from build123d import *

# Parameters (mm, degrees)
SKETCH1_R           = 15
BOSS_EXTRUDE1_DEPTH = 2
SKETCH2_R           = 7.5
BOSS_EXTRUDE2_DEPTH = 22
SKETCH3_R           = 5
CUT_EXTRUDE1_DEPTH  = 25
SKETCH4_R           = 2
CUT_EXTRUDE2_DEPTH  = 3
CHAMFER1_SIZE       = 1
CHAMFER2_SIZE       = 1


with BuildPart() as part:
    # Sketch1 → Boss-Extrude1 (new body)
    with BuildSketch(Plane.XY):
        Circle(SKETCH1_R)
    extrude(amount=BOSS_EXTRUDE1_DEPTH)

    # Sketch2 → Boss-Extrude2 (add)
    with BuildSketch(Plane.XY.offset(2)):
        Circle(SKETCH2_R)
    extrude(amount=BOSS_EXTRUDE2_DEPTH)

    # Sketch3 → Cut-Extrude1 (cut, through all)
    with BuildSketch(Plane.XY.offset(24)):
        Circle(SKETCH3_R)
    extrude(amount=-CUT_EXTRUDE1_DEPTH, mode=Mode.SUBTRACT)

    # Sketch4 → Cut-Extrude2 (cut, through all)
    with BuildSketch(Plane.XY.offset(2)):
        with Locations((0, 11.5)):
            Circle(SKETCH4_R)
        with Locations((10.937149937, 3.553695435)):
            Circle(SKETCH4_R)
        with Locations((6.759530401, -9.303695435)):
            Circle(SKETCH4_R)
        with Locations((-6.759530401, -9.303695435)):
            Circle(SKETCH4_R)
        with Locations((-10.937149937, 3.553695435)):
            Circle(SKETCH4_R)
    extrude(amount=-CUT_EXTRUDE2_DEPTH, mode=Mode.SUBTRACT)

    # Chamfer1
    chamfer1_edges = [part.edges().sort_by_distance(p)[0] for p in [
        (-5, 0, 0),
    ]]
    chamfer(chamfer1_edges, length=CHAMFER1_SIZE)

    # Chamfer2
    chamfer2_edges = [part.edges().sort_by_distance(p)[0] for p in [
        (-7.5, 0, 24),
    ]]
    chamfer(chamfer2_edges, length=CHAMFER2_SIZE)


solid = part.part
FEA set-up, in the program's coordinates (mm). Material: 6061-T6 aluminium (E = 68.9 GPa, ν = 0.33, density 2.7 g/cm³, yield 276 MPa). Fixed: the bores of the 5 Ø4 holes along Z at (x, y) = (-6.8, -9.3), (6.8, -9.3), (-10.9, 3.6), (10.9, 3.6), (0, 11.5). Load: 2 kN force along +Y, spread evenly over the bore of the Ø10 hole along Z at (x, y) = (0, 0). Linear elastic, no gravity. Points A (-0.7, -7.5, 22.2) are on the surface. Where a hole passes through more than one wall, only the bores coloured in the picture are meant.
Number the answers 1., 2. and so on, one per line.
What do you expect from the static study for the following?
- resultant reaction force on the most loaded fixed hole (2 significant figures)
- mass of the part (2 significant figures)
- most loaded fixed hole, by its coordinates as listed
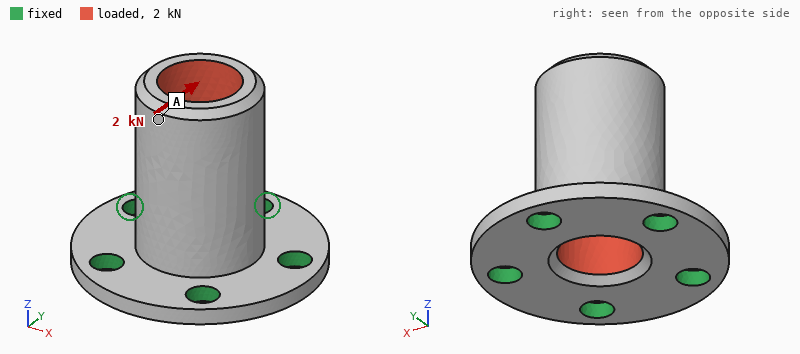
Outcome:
1. 1.2 kN
2. 8.8 g
3. (0, 11.5)
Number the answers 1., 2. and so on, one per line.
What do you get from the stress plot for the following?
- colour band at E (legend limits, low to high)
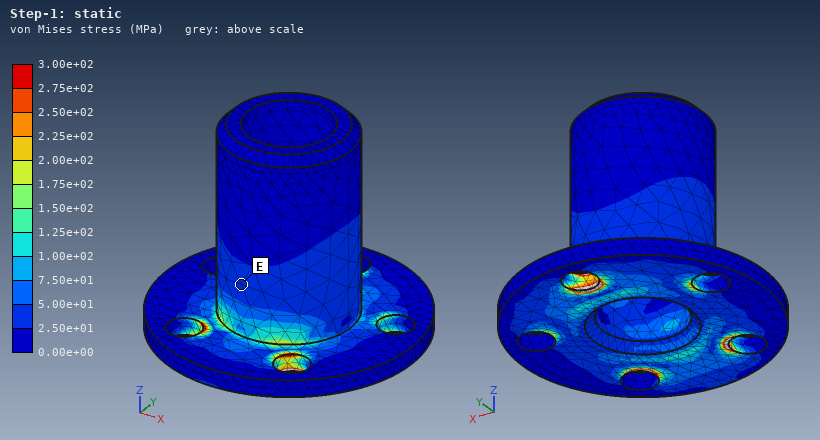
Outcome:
1. 2.50e+01 to 5.00e+01 MPa
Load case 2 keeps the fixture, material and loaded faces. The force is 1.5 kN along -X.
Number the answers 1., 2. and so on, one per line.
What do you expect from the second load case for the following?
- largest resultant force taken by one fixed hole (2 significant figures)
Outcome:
1. 850 N
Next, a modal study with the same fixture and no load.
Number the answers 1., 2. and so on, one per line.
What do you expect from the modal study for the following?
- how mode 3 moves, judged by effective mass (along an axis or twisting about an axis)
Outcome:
1. along Z
